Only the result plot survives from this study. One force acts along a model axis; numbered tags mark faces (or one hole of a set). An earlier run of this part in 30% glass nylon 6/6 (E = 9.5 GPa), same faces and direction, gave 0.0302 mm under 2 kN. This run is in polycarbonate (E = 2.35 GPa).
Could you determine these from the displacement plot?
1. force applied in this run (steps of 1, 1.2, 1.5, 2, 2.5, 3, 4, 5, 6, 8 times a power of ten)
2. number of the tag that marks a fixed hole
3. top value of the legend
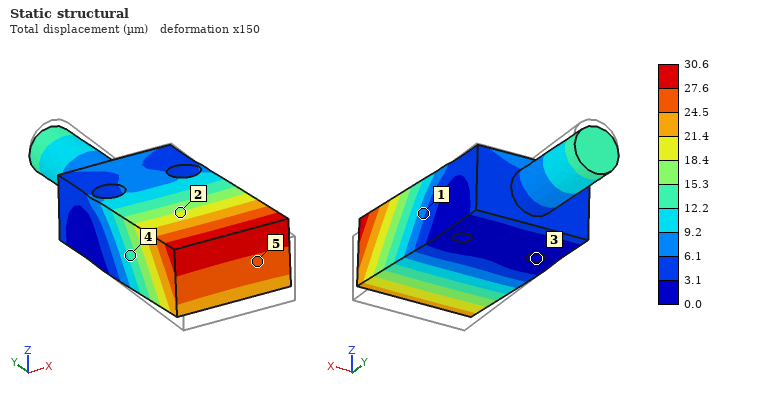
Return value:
500 N
3
30.6 µm
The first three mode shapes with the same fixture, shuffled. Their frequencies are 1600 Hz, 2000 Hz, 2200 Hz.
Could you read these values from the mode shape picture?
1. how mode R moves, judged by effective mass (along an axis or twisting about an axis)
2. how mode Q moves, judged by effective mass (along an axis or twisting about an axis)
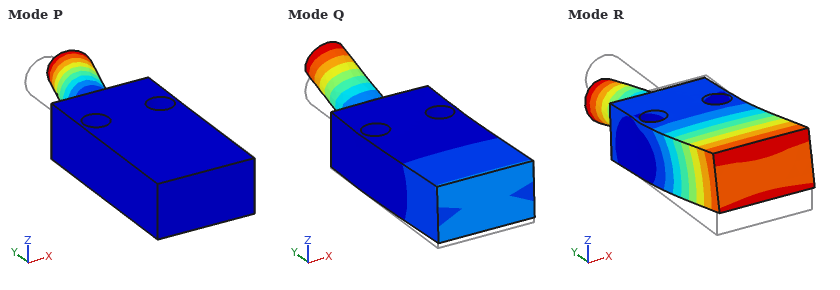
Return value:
along Z
along Z
